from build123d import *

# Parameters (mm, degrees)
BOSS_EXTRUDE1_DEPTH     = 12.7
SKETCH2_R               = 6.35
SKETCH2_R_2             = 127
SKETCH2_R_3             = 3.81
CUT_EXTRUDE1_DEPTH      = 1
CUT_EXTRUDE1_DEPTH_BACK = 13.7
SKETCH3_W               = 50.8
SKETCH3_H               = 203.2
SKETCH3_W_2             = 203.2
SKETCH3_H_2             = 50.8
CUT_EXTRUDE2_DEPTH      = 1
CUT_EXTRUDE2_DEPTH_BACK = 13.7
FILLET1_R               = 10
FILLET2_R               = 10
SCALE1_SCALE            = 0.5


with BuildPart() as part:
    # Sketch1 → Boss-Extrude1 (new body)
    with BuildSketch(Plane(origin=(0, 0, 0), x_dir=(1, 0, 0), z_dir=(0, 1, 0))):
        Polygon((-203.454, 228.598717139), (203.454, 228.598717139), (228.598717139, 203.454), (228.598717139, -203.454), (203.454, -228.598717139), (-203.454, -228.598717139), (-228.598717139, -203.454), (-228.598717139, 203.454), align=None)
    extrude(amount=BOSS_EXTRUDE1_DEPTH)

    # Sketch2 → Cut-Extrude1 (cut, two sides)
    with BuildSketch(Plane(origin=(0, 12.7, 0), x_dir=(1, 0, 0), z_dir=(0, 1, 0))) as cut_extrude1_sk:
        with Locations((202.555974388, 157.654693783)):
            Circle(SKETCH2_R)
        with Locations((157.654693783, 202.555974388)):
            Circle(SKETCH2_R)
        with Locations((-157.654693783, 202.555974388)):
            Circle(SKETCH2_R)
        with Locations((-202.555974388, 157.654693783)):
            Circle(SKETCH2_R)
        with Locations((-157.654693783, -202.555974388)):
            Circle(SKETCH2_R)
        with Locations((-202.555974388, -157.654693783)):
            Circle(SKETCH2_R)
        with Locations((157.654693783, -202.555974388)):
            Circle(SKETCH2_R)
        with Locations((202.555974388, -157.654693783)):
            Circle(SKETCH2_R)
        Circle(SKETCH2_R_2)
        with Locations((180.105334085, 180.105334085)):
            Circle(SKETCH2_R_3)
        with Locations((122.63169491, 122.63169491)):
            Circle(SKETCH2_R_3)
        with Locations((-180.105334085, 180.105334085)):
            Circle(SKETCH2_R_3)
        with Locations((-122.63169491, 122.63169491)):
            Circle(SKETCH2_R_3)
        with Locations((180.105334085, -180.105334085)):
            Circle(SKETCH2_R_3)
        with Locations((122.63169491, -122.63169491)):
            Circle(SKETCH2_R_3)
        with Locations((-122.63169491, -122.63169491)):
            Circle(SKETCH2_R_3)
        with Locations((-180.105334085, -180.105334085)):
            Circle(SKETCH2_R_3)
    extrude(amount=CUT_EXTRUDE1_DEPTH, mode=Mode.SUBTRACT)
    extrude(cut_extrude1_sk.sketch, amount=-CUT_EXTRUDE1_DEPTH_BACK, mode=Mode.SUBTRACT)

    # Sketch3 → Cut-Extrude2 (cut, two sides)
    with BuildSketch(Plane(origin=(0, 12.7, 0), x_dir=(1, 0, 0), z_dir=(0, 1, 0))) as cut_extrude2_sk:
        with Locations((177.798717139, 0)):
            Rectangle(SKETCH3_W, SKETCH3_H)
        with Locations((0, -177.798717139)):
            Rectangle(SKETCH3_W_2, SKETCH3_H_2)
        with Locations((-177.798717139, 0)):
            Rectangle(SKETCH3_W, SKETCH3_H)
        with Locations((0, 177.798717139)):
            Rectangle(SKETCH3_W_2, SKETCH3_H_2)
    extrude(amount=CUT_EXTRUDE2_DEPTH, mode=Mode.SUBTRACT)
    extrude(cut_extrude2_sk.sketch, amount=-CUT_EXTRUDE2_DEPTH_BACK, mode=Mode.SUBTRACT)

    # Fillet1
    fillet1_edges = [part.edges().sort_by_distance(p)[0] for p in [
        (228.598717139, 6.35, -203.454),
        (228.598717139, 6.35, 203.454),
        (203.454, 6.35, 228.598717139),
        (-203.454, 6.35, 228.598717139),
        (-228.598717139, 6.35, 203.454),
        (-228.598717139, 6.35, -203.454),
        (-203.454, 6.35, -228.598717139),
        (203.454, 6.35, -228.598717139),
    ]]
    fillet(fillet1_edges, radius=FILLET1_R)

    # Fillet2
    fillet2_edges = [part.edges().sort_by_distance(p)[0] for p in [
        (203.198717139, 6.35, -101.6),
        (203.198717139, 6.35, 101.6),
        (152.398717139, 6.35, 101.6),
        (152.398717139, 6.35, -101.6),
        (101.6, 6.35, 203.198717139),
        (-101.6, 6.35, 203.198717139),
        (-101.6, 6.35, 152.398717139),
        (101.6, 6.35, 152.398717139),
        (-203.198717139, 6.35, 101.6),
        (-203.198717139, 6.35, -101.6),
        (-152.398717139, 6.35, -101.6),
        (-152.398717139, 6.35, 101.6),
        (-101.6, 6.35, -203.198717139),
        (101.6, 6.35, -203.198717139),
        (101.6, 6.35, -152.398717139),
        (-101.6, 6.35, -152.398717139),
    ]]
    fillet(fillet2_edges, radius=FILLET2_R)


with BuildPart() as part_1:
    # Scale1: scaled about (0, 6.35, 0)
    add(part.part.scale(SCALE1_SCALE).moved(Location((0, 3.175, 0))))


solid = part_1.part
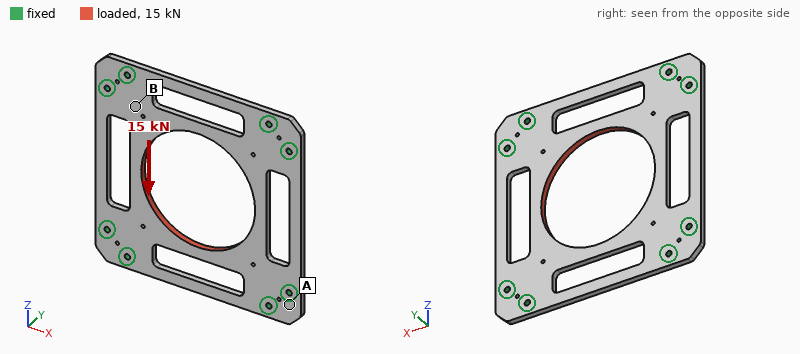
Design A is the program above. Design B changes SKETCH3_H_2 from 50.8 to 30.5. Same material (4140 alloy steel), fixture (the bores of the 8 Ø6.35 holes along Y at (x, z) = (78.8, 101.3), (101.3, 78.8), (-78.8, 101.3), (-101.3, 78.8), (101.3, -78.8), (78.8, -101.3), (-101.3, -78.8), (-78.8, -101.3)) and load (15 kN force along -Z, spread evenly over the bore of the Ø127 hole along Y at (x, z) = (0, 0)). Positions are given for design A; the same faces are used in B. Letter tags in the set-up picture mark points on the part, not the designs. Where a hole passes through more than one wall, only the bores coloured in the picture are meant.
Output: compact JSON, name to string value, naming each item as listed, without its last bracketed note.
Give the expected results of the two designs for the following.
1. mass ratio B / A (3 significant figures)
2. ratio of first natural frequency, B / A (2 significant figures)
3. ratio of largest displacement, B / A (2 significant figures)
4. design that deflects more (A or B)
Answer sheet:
{"mass ratio B / A": "1.07", "ratio of first natural frequency, B / A": "0.98", "ratio of largest displacement, B / A": "0.73", "design that deflects more": "A"}
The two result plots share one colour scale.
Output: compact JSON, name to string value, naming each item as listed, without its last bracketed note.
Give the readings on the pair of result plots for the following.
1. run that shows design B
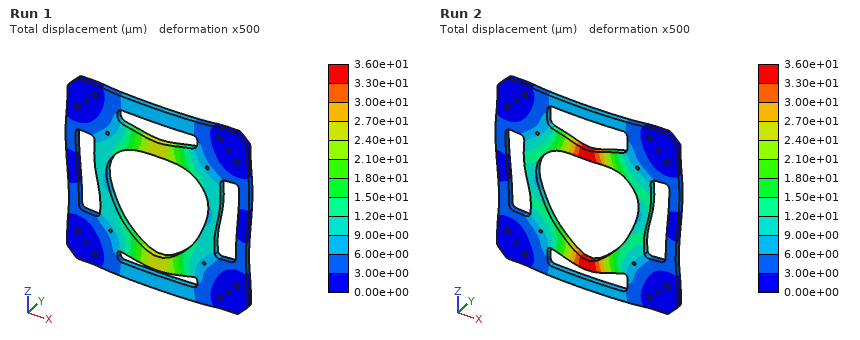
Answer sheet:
{"run that shows design B": "Run 1"}
